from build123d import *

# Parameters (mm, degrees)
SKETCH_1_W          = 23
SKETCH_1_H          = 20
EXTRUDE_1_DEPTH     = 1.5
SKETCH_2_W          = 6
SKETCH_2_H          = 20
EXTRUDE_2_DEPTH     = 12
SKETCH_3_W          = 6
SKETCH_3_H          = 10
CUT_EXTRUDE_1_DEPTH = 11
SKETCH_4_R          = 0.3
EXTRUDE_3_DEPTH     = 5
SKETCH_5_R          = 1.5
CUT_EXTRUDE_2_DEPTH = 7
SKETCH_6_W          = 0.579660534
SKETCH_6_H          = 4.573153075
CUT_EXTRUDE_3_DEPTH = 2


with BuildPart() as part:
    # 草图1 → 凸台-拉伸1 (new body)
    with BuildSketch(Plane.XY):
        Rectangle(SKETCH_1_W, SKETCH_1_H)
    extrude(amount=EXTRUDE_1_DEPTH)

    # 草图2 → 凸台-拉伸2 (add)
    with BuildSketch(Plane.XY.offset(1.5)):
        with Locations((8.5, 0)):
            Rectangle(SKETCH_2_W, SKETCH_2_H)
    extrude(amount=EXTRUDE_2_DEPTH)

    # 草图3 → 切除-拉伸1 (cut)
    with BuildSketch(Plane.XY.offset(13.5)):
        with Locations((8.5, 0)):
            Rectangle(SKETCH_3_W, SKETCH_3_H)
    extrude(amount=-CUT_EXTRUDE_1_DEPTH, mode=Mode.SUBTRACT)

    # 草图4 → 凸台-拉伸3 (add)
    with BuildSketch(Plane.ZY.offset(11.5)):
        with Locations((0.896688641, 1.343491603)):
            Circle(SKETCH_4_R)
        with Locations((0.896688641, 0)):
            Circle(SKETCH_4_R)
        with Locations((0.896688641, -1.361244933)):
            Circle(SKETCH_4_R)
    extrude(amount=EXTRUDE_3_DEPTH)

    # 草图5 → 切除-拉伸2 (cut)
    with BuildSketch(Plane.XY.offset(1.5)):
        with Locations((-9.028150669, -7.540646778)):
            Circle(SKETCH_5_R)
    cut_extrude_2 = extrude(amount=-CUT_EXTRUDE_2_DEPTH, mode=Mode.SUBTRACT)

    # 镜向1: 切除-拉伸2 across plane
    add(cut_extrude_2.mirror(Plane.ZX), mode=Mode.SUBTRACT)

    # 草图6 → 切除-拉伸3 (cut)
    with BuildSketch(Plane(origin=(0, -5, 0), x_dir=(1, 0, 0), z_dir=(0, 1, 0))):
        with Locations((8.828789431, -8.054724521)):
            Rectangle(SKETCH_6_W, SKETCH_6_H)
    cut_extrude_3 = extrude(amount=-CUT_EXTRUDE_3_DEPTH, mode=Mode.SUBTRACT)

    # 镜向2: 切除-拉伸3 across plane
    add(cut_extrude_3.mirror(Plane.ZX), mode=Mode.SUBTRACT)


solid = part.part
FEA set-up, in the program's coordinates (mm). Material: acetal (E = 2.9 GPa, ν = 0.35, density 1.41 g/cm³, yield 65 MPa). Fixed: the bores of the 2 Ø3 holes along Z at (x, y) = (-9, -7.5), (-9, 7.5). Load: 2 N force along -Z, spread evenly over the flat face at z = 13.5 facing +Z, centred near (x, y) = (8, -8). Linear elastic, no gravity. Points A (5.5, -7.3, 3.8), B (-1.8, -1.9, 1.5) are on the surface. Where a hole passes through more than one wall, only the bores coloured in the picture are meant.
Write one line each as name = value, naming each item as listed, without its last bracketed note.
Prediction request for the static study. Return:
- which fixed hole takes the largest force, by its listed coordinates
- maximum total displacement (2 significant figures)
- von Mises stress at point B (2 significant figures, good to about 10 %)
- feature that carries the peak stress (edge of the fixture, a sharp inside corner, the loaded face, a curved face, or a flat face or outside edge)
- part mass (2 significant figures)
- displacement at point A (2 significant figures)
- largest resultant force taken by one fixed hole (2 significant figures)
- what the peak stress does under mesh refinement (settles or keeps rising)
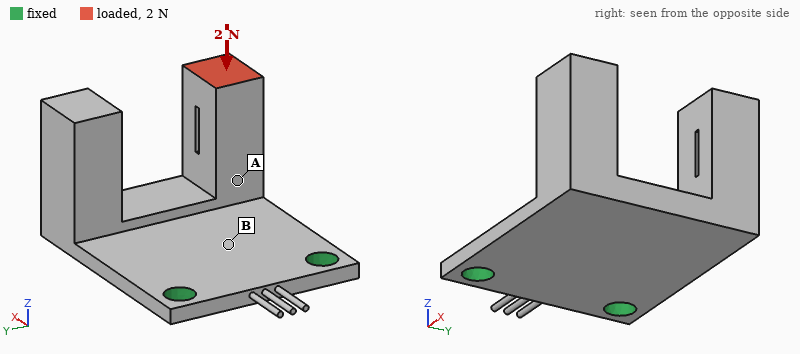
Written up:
which fixed hole takes the largest force, by its listed coordinates = (-9, -7.5)
maximum total displacement = 0.38 mm
von Mises stress at point B = 2.7 MPa
feature that carries the peak stress = edge of the fixture
part mass = 2.0 g
displacement at point A = 0.18 mm
largest resultant force taken by one fixed hole = 2.0 N
what the peak stress does under mesh refinement = keeps rising
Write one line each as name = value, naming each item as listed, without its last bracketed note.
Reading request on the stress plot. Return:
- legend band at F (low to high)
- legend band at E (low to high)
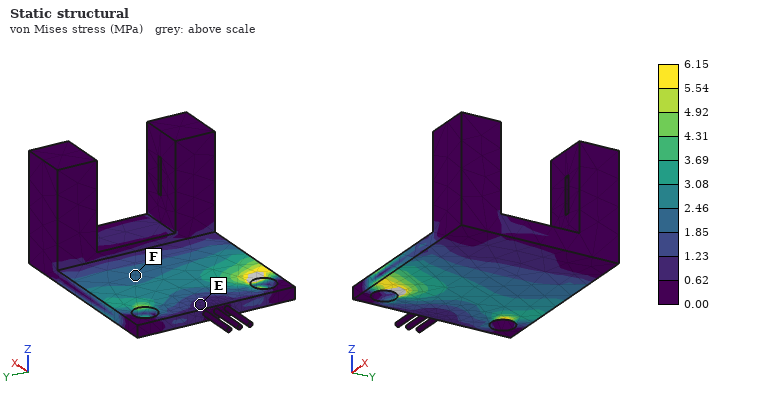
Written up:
legend band at F = 1.85 to 2.46 MPa
legend band at E = 0.62 to 1.23 MPa
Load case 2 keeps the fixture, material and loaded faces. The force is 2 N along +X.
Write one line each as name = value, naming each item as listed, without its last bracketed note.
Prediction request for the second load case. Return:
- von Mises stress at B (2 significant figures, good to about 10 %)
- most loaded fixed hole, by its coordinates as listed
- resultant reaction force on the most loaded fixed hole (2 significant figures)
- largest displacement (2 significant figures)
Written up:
von Mises stress at B = 3.1 MPa
most loaded fixed hole, by its coordinates as listed = (-9, -7.5)
resultant reaction force on the most loaded fixed hole = 2.0 N
largest displacement = 0.44 mm
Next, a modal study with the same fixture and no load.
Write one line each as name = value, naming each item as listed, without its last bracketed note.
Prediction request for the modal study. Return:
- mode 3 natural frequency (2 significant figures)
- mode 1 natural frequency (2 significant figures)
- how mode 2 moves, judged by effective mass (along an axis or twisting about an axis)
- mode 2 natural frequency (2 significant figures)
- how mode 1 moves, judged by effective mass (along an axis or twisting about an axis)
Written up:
mode 3 natural frequency = 1700 Hz
mode 1 natural frequency = 370 Hz
how mode 2 moves, judged by effective mass = along Y
mode 2 natural frequency = 790 Hz
how mode 1 moves, judged by effective mass = along Z
